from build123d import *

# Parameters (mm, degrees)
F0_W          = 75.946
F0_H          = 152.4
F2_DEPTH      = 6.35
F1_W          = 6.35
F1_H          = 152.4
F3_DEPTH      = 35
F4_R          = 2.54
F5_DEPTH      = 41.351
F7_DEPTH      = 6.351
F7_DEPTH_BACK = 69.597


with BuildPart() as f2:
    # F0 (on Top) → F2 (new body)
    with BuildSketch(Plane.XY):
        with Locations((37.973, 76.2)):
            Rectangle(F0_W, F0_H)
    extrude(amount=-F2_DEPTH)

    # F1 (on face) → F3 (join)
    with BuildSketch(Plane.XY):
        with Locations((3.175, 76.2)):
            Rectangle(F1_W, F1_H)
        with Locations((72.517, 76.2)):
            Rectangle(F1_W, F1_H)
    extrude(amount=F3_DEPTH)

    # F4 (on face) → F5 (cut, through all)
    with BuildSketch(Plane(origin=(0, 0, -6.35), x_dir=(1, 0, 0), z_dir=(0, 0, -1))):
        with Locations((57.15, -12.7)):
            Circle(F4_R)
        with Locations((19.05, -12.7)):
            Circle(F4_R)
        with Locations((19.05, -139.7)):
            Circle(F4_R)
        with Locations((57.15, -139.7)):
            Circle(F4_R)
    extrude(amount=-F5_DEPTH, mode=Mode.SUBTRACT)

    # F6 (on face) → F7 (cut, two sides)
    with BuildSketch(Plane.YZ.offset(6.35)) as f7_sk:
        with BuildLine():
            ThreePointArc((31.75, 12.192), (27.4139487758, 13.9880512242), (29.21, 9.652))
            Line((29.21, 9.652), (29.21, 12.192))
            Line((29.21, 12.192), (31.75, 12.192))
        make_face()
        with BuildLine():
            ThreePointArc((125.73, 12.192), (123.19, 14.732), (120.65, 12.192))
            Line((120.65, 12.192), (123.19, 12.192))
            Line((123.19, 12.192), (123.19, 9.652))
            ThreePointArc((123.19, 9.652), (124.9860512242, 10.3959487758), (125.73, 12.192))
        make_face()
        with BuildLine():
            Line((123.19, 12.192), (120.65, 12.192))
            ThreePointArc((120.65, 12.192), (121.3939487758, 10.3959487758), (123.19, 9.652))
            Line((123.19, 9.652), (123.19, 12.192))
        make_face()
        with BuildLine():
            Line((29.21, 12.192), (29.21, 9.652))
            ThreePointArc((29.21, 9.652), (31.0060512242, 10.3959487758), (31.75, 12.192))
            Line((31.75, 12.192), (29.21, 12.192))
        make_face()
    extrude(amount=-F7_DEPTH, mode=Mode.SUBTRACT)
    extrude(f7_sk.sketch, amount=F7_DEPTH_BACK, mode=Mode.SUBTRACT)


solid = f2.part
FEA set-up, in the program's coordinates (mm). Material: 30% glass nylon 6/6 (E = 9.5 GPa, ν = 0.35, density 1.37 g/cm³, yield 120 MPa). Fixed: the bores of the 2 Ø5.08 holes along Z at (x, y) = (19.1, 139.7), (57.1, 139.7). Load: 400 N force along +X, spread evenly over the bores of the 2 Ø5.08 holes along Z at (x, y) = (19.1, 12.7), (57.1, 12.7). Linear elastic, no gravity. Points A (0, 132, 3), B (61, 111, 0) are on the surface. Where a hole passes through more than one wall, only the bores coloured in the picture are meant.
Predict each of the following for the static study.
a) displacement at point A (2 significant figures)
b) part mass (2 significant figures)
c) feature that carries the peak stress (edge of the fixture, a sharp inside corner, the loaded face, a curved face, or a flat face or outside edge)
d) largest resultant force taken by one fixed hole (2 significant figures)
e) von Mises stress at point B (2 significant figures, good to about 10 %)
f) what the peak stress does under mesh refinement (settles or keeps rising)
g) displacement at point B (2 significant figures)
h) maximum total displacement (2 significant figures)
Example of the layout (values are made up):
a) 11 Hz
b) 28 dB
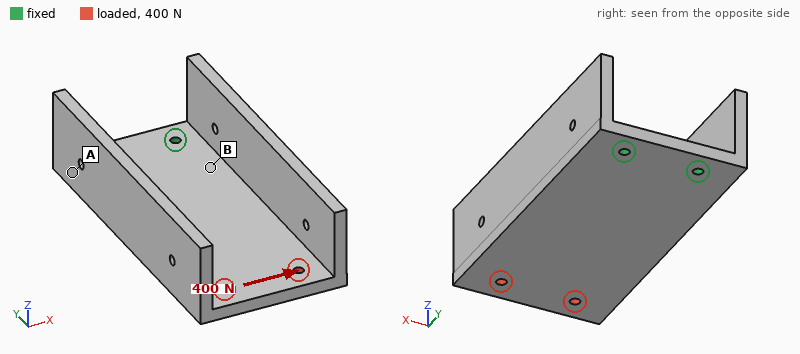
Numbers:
a) 0.042 mm
b) 190 g
c) edge of the fixture
d) 1.3 kN
e) 3.4 MPa
f) keeps rising
g) 0.044 mm
h) 0.24 mm
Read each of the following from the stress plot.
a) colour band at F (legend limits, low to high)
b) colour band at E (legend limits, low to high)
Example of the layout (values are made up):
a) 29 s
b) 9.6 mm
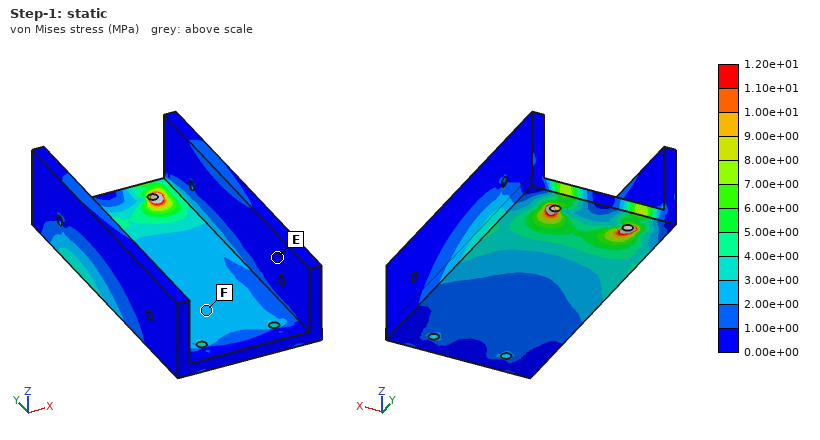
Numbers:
a) 2.00e+00 to 3.00e+00 MPa
b) 0.00e+00 to 1.00e+00 MPa
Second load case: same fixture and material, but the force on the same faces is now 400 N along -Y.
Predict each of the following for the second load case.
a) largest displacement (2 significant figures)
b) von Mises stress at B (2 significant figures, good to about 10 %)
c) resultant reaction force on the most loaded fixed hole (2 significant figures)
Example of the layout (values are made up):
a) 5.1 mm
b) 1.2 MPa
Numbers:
a) 24 µm
b) 0.75 MPa
c) 200 N
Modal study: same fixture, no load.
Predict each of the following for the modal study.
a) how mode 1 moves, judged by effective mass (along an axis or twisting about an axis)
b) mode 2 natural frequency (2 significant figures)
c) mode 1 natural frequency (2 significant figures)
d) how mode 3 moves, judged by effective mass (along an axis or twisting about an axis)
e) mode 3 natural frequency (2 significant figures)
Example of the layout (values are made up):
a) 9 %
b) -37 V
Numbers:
a) along Z
b) 330 Hz
c) 180 Hz
d) along X
e) 800 Hz
